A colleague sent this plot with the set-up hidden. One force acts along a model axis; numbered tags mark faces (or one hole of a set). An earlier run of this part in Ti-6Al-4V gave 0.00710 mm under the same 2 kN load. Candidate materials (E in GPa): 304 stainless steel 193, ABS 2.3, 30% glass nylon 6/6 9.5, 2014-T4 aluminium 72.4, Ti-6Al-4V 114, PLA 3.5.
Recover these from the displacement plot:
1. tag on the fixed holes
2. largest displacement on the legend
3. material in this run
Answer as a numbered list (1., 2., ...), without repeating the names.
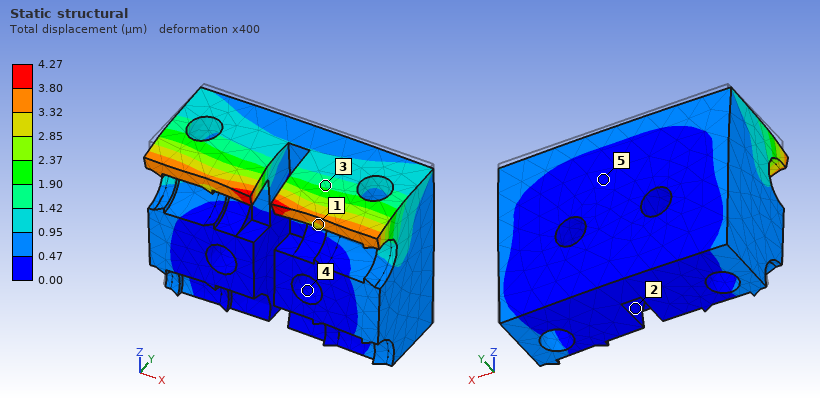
1. 4
2. 4.27 µm
3. 304 stainless steel
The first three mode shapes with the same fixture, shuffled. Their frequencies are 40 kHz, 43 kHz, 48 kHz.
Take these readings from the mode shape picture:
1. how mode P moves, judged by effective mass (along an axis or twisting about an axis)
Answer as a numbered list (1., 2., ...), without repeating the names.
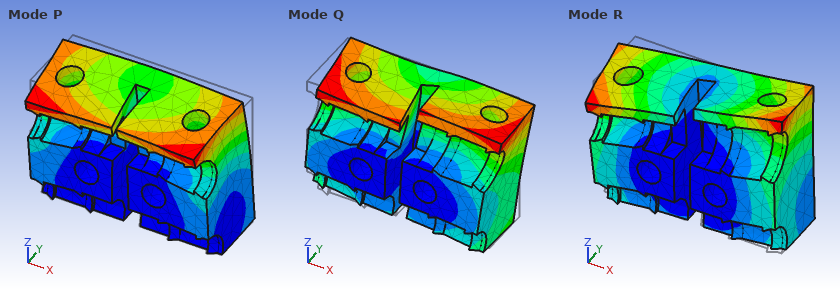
1. along Y
